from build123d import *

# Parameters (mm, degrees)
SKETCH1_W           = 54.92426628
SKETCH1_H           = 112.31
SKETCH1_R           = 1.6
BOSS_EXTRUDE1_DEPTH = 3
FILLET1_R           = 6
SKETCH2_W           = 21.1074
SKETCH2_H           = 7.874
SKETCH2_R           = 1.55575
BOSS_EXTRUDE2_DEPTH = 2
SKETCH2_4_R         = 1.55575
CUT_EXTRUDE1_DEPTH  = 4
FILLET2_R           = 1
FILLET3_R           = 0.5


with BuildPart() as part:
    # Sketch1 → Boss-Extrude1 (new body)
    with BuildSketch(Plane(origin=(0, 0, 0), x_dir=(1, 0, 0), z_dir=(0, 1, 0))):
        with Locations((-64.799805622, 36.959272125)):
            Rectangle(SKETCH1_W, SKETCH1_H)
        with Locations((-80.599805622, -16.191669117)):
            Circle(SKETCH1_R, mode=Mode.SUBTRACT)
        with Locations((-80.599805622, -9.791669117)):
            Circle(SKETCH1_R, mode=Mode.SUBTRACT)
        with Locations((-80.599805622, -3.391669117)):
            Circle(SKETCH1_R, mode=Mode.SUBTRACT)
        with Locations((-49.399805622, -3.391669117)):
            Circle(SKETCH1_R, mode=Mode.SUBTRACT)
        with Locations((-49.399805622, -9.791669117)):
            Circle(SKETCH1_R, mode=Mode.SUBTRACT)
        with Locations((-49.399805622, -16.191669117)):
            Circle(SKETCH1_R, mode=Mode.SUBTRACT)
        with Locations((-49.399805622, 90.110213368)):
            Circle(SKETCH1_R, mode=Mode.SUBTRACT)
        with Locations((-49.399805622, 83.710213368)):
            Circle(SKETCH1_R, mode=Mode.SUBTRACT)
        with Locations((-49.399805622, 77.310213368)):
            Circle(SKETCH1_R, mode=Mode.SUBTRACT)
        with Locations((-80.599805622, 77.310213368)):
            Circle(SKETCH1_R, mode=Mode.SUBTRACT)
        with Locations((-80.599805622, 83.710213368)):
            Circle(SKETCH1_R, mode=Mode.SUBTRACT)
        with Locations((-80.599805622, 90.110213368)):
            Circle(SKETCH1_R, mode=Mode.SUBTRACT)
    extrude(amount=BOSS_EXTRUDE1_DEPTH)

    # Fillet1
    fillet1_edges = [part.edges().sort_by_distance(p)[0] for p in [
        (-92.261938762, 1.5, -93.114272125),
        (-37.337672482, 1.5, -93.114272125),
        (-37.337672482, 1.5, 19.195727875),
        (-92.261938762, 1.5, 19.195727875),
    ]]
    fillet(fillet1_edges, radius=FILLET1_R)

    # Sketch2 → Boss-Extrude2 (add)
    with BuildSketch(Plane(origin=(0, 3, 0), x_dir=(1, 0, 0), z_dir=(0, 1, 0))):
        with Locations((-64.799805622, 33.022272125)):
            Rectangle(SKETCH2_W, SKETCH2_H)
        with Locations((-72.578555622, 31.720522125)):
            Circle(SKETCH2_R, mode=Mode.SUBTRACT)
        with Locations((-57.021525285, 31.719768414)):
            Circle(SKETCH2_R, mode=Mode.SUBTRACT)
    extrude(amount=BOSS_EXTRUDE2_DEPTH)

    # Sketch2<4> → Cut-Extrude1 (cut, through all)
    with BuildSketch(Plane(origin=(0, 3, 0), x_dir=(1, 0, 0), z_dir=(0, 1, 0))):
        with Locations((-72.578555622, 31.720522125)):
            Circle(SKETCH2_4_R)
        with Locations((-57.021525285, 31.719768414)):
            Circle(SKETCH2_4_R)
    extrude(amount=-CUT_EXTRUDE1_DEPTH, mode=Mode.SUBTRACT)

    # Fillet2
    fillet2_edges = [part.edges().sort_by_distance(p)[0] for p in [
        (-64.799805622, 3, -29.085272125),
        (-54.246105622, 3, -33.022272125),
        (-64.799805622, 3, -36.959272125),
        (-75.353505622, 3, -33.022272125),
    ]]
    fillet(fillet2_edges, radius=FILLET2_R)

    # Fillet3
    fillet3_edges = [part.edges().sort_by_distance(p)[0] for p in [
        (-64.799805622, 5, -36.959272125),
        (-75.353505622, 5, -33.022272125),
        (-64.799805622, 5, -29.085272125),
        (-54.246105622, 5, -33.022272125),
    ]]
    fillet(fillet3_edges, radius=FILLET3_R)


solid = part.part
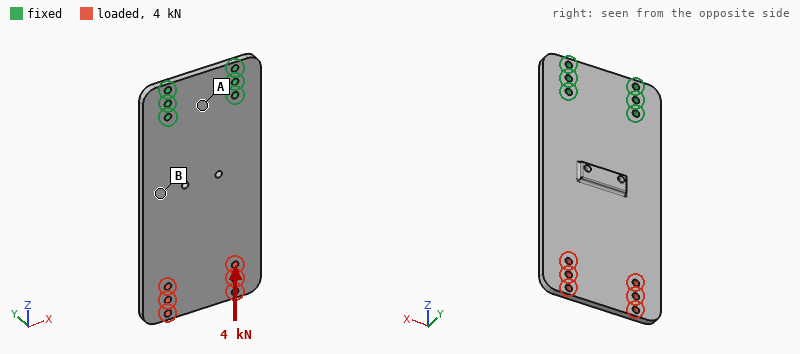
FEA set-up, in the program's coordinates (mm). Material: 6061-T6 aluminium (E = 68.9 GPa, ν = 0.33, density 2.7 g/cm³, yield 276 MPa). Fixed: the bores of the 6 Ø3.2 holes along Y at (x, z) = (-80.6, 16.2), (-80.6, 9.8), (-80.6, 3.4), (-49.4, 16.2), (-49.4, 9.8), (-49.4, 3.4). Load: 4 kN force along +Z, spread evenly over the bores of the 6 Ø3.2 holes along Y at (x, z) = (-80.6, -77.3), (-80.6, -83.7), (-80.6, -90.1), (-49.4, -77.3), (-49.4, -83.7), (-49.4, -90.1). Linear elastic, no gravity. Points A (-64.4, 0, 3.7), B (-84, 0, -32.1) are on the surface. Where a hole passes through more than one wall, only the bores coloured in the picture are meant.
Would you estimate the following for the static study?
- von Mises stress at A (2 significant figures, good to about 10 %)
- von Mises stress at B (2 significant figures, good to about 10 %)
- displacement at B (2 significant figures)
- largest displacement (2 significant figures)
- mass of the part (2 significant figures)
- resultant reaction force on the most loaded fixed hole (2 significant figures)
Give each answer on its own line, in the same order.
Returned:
10 MPa
28 MPa
16 µm
50 µm
50 g
1.3 kN
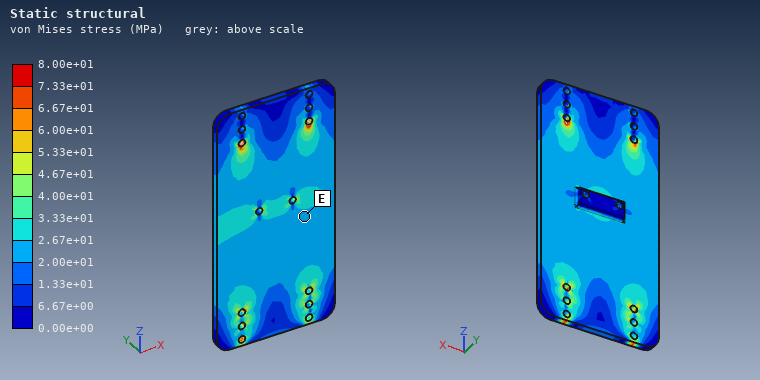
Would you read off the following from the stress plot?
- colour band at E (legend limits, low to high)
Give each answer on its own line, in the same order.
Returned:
2.00e+01 to 2.67e+01 MPa
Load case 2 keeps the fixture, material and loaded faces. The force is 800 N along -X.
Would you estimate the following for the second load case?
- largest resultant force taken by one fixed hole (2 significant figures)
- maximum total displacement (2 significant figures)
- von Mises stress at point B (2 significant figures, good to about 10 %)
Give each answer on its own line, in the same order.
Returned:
1.4 kN
0.11 mm
20 MPa
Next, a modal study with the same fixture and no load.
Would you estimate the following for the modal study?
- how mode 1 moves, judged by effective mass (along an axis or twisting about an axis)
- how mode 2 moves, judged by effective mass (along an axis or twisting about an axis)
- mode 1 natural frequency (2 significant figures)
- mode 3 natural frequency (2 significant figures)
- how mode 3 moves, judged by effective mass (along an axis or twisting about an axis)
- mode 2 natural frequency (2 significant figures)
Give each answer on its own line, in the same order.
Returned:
along Y
twisting about Z
270 Hz
1700 Hz
along Y
1100 Hz
